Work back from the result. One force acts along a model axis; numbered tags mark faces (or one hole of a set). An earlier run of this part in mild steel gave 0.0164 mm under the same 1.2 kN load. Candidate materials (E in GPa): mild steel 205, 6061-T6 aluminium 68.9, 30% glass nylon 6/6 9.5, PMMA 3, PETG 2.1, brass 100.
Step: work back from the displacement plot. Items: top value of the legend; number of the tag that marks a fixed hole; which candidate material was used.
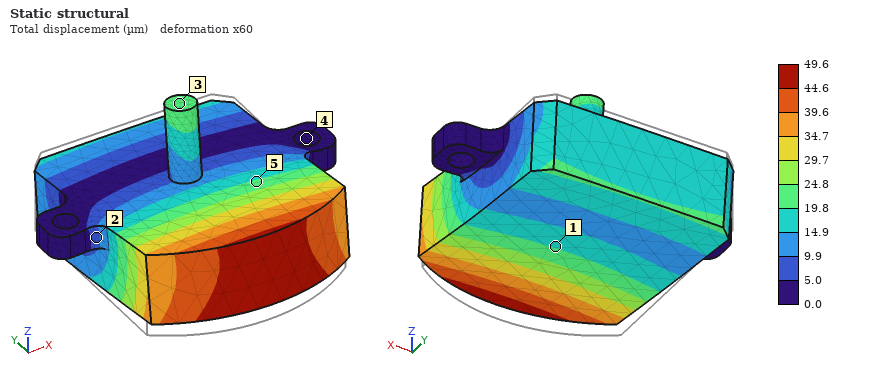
49.6 µm
4
6061-T6 aluminium
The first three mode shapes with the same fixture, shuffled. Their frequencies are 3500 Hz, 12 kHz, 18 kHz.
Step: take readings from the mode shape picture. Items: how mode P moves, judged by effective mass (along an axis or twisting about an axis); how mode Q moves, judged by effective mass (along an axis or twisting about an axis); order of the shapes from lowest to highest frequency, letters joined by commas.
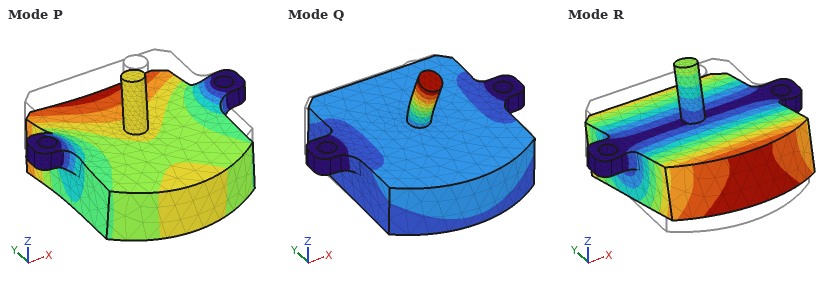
along Z
along Y
R, P, Q
